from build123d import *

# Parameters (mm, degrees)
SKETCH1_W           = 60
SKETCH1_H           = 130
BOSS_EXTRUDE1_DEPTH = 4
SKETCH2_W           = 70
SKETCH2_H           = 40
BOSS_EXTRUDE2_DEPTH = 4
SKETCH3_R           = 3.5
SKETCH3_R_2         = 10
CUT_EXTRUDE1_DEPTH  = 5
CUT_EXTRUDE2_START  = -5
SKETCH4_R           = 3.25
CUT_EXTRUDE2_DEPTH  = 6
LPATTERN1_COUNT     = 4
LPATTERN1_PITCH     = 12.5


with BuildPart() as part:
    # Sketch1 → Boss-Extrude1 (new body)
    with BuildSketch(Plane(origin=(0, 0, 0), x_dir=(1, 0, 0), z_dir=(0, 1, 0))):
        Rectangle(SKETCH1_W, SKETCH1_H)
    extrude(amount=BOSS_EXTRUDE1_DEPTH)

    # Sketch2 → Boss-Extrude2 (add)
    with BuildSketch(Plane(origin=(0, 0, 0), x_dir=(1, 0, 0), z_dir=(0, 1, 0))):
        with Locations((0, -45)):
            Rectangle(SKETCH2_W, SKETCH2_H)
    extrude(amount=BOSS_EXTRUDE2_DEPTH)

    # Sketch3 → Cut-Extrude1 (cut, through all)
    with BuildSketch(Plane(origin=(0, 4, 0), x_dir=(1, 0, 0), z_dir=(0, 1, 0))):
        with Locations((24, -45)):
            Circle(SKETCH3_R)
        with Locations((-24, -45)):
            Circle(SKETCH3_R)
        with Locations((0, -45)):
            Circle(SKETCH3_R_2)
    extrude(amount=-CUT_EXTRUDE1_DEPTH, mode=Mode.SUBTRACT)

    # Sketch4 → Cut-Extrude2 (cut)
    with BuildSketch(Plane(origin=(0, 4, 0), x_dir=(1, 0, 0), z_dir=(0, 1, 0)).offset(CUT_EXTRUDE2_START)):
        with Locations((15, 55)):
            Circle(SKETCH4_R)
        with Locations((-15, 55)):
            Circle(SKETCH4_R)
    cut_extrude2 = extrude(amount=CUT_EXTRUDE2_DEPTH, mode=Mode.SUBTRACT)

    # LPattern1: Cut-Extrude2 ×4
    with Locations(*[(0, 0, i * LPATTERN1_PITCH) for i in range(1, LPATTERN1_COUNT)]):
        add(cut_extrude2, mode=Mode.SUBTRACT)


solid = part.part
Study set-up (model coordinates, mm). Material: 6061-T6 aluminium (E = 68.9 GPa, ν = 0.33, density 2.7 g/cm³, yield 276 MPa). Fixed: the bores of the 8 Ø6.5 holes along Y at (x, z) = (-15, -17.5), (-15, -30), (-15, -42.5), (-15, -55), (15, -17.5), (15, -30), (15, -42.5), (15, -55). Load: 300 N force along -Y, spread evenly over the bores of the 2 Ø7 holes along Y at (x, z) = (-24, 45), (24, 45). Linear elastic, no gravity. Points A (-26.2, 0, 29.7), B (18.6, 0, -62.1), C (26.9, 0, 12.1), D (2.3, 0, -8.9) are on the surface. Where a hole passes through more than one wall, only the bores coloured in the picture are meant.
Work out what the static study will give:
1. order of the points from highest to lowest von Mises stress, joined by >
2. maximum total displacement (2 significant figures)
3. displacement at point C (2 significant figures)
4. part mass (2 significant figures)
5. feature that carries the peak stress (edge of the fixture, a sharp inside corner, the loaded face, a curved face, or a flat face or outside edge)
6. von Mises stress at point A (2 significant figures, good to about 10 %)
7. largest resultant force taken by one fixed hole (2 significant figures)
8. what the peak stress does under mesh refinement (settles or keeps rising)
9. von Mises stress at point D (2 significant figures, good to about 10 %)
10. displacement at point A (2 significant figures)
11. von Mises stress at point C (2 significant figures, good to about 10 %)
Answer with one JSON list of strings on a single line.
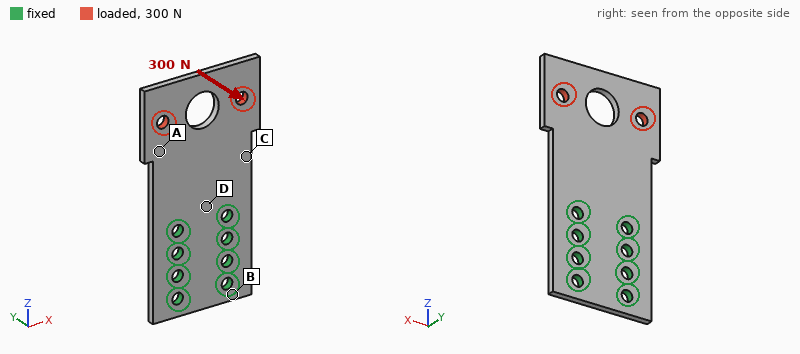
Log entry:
["D > C > A > B", "1.5 mm", "0.27 mm", "81 g", "edge of the fixture", "27 MPa", "350 N", "keeps rising", "84 MPa", "0.64 mm", "64 MPa"]
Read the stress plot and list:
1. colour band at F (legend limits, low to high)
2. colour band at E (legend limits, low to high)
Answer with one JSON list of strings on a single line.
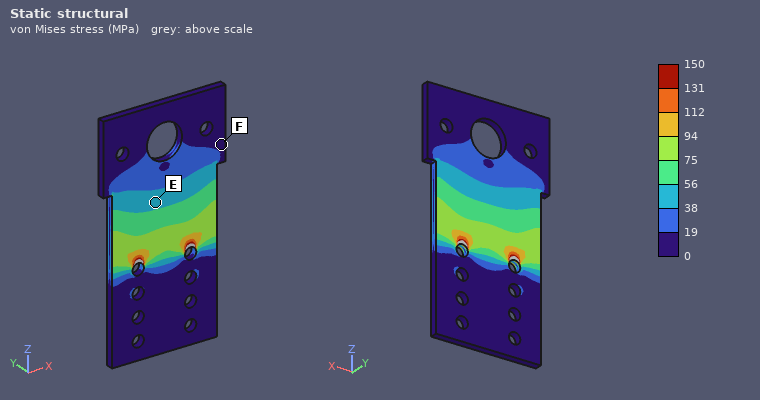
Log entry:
["0 to 19 MPa", "38 to 56 MPa"]
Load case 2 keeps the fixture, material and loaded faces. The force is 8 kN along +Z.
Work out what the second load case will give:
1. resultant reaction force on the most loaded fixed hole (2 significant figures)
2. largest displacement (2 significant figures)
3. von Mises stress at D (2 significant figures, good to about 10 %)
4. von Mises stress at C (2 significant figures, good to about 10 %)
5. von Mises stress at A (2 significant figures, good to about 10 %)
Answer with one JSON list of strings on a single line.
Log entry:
["3.0 kN", "42 µm", "22 MPa", "40 MPa", "46 MPa"]
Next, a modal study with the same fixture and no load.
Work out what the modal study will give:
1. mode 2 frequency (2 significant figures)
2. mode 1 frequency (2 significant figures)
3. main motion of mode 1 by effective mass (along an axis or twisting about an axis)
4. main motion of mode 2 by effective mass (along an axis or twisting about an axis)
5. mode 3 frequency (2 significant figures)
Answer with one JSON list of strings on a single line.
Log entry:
["1200 Hz", "500 Hz", "along Y", "twisting about Z", "2800 Hz"]
